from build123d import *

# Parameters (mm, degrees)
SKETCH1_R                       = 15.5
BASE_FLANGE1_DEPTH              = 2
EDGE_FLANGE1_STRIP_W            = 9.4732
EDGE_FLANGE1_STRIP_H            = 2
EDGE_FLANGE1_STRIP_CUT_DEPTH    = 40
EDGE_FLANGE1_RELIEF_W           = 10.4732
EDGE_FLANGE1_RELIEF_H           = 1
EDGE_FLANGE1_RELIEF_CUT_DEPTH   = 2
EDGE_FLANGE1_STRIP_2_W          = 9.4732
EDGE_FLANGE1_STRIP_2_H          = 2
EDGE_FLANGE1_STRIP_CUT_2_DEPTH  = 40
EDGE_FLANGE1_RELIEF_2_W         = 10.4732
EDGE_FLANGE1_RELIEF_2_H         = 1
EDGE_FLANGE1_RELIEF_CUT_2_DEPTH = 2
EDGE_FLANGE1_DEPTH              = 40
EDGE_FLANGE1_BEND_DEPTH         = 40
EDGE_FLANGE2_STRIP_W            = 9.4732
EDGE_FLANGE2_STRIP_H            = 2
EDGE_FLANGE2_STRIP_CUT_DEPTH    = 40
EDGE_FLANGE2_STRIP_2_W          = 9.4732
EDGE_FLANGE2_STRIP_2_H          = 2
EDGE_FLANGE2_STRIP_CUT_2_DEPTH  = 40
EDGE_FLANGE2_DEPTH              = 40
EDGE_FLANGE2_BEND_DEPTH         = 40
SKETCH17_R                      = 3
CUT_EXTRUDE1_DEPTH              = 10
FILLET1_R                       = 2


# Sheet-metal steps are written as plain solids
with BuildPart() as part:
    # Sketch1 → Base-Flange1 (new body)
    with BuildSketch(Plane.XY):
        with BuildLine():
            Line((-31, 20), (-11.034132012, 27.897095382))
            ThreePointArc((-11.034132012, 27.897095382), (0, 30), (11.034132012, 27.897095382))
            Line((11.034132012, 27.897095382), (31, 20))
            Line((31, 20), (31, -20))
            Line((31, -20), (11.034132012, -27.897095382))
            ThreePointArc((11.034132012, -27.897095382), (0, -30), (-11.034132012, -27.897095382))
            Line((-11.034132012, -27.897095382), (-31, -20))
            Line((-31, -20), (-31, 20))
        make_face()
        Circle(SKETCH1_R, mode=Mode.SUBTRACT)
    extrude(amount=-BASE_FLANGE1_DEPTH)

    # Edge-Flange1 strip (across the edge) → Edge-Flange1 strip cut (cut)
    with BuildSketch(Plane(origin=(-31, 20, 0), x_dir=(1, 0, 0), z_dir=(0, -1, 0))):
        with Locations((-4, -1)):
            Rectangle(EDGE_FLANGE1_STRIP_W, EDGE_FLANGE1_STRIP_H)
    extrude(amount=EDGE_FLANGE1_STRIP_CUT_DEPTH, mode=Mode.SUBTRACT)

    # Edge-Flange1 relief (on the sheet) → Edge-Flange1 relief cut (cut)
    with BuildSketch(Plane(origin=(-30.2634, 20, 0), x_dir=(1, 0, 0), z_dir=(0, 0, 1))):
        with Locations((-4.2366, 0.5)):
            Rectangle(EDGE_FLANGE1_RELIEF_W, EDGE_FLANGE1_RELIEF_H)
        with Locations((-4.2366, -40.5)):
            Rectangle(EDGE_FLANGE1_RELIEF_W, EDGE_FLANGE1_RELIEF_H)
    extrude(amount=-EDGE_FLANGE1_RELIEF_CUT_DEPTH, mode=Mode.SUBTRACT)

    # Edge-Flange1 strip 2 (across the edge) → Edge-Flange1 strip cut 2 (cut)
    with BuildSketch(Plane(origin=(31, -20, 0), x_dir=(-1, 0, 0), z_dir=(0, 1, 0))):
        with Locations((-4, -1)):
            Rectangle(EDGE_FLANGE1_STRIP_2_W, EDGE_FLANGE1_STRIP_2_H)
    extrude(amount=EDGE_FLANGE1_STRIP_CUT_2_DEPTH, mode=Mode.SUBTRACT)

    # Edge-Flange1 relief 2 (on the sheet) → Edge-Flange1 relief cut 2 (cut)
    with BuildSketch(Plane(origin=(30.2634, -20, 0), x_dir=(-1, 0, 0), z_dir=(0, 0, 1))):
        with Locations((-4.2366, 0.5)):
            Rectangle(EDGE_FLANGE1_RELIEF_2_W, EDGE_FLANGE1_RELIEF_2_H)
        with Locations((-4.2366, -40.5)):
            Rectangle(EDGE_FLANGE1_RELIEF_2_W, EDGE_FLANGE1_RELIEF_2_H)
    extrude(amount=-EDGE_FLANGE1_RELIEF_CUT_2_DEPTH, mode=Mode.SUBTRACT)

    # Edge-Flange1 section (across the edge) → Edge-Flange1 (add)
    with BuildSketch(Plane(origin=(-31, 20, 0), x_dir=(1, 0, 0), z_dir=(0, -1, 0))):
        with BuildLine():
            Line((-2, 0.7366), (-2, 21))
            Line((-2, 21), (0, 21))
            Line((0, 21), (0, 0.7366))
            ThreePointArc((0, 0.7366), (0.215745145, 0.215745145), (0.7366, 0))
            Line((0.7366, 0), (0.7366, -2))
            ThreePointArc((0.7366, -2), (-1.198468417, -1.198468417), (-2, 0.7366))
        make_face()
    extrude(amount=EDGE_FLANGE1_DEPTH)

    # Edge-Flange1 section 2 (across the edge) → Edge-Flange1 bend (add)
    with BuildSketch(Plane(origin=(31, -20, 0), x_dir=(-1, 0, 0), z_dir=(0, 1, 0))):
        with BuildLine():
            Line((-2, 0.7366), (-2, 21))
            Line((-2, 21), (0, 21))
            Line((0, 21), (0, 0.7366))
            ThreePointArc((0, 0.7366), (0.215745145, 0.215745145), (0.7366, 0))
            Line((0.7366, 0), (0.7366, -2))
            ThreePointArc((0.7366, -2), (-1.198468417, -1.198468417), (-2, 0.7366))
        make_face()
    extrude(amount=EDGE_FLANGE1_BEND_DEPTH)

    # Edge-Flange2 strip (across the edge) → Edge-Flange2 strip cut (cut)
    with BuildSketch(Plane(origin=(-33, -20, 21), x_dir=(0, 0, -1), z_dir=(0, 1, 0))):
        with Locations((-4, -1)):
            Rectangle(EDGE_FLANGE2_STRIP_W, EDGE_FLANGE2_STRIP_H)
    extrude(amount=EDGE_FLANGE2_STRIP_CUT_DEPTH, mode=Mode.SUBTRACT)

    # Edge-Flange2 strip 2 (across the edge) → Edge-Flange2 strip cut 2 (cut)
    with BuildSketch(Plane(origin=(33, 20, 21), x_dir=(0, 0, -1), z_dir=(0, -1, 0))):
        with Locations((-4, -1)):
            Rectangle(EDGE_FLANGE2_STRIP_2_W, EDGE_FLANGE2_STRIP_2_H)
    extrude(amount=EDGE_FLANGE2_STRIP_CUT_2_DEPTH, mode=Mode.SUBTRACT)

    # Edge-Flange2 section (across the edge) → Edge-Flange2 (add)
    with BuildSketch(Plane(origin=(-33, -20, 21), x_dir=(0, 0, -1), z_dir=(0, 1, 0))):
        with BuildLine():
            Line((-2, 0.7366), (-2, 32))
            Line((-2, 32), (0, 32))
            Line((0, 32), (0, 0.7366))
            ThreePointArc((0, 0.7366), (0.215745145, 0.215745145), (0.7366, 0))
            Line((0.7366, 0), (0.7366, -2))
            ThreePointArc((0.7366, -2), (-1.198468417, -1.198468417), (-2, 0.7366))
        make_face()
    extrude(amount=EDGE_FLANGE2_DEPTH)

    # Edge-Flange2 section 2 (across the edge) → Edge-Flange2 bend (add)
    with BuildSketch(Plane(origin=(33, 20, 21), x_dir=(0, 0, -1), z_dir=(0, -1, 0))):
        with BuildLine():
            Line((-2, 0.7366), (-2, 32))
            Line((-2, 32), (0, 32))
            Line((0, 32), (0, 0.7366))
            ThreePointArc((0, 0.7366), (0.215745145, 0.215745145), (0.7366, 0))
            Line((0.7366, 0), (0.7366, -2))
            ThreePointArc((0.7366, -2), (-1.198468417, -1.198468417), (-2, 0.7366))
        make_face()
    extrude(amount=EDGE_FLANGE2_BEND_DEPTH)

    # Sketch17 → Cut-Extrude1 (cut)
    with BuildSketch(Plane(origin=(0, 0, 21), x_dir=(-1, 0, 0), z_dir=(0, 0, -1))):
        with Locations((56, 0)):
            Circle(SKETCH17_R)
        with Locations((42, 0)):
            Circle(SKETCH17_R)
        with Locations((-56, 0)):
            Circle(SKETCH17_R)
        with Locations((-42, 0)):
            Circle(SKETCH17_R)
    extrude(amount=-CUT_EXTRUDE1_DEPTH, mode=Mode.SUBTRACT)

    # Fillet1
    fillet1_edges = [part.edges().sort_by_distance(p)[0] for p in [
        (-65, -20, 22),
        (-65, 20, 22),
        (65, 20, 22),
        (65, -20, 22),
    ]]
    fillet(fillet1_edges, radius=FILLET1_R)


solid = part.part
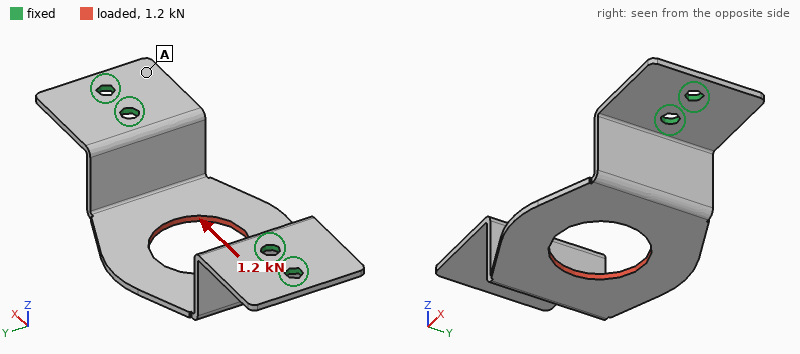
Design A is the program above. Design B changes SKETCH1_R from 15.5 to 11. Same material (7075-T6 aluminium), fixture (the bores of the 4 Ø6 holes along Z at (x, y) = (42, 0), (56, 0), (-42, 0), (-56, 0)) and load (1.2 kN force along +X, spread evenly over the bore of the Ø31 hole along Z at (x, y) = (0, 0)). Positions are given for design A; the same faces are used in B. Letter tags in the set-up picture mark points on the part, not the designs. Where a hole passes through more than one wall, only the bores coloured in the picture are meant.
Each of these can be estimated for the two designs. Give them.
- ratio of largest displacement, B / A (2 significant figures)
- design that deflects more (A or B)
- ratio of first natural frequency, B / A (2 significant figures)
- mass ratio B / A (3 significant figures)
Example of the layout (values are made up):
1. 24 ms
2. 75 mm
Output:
1. 0.90
2. A
3. 0.96
4. 1.06
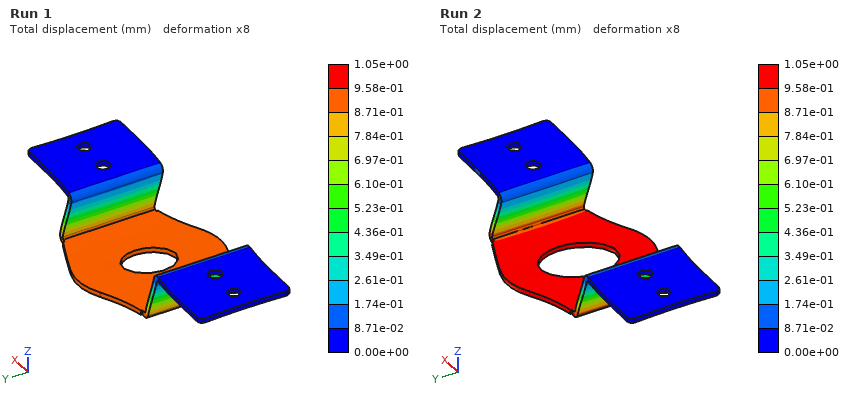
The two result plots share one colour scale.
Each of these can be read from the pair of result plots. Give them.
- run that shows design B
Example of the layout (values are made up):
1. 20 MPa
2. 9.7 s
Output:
1. Run 1
